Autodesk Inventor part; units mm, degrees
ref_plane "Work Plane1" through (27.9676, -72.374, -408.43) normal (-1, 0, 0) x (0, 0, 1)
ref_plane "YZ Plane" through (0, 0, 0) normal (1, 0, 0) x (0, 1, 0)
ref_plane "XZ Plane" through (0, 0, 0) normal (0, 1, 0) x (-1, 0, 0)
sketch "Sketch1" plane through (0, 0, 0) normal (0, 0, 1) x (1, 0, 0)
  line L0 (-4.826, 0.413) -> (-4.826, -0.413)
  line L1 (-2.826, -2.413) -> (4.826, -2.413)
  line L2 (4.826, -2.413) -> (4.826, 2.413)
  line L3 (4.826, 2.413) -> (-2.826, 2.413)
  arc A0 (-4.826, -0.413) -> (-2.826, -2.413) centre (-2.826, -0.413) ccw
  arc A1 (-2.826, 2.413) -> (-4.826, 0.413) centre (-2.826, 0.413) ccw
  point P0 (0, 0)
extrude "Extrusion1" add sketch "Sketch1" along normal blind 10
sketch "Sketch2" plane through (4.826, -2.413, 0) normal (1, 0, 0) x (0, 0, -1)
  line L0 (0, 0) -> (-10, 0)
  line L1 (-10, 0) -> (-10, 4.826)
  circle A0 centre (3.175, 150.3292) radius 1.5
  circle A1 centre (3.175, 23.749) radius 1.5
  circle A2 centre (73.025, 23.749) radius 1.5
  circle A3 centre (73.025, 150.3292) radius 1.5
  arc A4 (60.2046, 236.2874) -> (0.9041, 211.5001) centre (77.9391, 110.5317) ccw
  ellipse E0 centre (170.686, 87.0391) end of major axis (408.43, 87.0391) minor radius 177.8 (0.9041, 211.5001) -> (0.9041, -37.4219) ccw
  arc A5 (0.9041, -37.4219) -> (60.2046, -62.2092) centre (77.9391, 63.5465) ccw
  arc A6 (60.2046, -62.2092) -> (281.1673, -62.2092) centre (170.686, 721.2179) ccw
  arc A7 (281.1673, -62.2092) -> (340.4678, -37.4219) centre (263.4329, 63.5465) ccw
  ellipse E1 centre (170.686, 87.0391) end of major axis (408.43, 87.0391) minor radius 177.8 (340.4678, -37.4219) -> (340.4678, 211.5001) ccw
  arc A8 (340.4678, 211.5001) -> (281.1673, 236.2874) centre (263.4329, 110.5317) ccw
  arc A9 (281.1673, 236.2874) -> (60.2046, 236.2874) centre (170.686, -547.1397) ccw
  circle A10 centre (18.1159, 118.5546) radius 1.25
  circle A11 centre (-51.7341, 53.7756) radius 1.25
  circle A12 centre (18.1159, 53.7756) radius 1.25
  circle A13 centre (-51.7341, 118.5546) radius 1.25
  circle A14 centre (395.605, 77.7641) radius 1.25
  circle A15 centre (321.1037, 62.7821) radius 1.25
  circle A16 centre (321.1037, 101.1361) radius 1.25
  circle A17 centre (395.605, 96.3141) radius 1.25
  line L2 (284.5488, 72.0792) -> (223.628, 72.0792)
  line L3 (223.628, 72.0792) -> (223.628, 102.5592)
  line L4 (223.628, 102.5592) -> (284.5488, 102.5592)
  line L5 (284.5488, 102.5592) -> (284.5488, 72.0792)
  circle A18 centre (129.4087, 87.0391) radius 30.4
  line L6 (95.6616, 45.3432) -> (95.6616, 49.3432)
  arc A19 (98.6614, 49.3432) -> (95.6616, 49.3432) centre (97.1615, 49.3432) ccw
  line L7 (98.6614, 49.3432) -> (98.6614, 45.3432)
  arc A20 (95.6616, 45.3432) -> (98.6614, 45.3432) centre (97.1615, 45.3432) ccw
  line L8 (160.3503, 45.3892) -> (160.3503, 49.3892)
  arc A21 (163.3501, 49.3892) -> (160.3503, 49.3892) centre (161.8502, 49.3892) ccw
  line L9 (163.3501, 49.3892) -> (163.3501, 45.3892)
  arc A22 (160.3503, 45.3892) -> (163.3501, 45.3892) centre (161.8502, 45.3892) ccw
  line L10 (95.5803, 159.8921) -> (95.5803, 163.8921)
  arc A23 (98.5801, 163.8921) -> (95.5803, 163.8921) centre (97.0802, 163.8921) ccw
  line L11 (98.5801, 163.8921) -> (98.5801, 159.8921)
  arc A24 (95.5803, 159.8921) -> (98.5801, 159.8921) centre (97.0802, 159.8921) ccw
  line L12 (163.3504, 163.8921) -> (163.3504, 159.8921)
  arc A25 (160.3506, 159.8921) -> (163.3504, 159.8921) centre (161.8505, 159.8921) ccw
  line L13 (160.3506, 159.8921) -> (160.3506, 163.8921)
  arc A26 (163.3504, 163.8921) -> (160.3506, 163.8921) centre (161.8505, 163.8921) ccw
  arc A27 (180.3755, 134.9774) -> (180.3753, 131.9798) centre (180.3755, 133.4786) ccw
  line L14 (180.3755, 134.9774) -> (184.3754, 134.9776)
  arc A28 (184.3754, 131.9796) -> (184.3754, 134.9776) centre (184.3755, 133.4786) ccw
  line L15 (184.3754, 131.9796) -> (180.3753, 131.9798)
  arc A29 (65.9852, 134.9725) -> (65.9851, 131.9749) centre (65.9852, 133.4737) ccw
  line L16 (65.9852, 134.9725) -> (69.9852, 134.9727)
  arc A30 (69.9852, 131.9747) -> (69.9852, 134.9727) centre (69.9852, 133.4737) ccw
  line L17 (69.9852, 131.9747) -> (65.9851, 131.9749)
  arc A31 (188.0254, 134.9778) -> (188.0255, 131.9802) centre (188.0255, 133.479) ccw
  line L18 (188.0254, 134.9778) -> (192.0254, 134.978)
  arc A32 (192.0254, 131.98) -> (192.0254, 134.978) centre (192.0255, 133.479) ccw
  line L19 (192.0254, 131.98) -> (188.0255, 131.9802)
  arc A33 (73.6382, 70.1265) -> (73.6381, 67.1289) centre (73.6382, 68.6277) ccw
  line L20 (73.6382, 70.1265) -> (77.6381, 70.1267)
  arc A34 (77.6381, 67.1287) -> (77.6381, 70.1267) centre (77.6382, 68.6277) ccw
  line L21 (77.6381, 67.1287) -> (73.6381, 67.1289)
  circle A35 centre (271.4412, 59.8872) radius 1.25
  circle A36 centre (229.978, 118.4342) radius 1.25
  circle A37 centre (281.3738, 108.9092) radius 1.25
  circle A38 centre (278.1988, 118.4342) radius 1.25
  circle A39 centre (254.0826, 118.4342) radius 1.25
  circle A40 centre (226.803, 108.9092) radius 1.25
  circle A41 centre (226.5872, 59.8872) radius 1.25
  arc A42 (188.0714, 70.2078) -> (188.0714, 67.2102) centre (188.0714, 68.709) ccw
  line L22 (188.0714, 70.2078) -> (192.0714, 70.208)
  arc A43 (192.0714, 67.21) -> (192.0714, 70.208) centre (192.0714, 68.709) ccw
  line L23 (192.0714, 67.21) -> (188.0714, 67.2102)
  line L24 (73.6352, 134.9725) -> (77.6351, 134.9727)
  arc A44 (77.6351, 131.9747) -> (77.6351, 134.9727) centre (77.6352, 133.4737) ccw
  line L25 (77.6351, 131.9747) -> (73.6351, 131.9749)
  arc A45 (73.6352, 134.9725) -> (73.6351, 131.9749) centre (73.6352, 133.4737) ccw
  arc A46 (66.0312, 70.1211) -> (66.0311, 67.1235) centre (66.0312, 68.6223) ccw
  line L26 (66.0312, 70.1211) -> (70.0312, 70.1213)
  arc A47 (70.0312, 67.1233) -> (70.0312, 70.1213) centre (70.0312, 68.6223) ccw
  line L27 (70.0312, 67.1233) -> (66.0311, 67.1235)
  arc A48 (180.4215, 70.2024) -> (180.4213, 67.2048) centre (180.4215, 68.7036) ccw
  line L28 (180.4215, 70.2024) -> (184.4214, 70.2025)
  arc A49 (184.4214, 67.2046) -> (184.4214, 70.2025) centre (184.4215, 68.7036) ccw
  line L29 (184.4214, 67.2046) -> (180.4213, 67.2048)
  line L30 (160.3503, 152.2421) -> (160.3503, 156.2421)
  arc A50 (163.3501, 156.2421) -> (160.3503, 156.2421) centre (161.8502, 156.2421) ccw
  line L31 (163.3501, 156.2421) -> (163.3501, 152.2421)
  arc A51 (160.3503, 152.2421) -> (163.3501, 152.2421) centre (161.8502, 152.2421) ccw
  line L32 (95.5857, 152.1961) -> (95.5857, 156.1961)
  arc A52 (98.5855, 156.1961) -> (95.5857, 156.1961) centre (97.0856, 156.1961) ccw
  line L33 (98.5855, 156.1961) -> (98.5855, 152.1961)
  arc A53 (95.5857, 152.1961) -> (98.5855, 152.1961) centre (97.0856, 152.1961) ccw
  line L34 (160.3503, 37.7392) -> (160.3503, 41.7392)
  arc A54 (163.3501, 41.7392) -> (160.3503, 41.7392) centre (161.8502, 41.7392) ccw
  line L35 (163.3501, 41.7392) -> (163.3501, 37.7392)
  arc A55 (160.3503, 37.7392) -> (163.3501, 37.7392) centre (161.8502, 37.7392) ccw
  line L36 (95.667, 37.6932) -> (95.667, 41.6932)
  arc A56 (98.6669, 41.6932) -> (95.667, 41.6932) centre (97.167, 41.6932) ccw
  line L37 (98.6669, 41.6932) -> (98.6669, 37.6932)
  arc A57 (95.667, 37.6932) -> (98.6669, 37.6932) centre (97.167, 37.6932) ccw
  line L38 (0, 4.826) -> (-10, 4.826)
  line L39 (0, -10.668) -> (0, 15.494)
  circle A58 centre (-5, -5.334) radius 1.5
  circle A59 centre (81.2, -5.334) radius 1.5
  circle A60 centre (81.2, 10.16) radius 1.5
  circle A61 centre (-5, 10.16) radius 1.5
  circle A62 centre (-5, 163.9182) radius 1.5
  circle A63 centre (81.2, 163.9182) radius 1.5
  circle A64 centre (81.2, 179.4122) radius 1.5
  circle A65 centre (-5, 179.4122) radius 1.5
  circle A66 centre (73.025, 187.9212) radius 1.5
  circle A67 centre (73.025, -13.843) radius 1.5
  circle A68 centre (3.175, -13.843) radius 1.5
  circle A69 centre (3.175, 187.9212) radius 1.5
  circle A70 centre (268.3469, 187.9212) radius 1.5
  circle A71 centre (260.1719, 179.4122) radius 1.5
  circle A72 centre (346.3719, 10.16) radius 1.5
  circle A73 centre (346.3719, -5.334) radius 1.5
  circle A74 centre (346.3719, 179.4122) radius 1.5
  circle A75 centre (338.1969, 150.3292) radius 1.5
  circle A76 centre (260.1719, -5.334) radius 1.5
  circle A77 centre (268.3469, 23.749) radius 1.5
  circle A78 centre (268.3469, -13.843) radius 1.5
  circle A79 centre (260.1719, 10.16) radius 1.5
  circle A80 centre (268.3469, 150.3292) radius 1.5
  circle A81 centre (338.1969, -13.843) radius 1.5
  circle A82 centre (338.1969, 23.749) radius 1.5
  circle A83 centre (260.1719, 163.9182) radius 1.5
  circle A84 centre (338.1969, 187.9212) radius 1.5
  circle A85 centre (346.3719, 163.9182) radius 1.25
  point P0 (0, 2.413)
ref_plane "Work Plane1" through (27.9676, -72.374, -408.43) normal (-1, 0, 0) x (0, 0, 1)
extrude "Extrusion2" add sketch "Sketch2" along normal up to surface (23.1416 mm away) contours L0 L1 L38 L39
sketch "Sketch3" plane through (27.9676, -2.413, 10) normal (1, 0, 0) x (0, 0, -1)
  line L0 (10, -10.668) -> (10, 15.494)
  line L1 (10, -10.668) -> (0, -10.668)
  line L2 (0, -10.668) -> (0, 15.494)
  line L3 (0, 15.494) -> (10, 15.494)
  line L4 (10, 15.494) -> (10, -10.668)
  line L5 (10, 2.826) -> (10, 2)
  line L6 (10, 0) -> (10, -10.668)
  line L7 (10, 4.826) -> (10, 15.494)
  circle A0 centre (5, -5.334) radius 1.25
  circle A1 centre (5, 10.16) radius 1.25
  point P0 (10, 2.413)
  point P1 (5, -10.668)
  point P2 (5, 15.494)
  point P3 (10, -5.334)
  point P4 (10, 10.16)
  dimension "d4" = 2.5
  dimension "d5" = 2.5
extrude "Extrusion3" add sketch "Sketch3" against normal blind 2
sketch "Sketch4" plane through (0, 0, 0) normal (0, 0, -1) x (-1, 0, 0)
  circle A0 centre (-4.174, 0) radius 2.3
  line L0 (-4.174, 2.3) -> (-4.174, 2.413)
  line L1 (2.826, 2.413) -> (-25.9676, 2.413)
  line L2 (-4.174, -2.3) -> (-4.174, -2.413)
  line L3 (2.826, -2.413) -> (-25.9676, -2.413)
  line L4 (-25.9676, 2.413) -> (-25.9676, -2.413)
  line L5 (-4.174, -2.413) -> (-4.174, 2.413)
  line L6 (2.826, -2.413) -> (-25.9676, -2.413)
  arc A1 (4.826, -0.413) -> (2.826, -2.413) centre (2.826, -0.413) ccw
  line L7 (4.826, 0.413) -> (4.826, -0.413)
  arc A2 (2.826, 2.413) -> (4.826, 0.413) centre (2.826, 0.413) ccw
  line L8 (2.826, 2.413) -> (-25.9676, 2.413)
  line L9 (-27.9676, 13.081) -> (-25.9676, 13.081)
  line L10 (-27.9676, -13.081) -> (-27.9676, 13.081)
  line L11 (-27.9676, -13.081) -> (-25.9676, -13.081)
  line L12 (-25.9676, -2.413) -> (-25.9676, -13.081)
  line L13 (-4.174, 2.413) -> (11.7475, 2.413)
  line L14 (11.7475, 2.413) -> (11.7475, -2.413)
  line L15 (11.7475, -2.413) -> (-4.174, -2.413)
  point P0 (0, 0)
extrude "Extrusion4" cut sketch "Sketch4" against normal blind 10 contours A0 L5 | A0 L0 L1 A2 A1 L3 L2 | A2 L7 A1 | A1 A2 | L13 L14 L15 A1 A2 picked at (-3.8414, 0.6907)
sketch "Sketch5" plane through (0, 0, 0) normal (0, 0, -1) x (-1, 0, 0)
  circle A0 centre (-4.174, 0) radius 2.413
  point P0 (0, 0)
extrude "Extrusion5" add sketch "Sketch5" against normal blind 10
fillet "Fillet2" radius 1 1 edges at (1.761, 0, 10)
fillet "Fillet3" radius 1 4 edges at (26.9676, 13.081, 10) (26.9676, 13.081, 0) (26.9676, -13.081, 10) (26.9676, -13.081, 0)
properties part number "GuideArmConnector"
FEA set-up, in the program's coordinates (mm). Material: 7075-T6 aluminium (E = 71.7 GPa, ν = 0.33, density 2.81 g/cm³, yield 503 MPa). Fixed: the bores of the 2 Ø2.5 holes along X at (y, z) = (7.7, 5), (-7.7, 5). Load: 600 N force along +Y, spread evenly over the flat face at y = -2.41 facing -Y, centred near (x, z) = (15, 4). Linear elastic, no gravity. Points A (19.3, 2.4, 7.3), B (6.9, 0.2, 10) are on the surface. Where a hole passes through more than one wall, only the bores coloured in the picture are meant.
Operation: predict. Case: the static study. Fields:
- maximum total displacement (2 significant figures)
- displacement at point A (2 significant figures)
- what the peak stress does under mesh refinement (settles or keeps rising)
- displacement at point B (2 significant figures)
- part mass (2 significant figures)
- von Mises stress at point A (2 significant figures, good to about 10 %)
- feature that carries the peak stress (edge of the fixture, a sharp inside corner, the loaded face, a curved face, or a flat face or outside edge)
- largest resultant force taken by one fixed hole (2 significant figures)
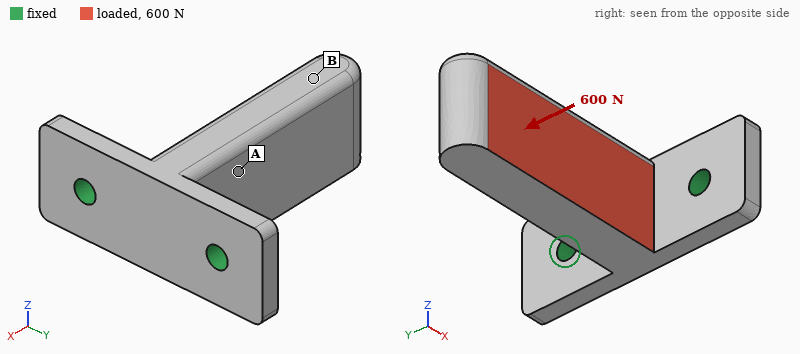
0.32 mm
0.081 mm
keeps rising
0.24 mm
4.6 g
83 MPa
edge of the fixture
730 N
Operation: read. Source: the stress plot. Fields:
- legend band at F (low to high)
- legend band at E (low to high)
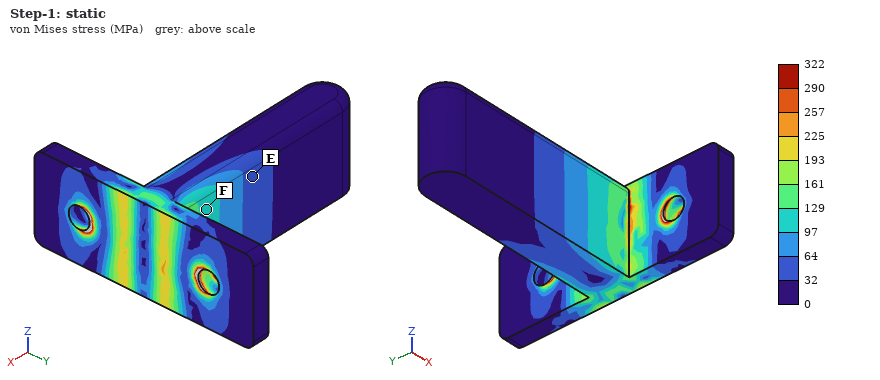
97 to 129 MPa
32 to 64 MPa
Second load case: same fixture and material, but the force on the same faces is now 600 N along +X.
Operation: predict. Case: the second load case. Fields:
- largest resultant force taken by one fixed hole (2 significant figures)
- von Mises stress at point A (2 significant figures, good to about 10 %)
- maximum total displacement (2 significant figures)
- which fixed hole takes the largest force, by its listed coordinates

440 N
19 MPa
85 µm
(-7.7, 5)
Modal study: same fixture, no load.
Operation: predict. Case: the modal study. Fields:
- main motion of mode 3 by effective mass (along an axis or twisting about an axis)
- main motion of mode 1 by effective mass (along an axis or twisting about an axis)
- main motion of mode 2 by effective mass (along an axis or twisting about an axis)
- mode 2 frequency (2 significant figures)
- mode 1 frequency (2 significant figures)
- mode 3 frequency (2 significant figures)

along X
along Z
along Y
4600 Hz
3400 Hz
16 kHz
